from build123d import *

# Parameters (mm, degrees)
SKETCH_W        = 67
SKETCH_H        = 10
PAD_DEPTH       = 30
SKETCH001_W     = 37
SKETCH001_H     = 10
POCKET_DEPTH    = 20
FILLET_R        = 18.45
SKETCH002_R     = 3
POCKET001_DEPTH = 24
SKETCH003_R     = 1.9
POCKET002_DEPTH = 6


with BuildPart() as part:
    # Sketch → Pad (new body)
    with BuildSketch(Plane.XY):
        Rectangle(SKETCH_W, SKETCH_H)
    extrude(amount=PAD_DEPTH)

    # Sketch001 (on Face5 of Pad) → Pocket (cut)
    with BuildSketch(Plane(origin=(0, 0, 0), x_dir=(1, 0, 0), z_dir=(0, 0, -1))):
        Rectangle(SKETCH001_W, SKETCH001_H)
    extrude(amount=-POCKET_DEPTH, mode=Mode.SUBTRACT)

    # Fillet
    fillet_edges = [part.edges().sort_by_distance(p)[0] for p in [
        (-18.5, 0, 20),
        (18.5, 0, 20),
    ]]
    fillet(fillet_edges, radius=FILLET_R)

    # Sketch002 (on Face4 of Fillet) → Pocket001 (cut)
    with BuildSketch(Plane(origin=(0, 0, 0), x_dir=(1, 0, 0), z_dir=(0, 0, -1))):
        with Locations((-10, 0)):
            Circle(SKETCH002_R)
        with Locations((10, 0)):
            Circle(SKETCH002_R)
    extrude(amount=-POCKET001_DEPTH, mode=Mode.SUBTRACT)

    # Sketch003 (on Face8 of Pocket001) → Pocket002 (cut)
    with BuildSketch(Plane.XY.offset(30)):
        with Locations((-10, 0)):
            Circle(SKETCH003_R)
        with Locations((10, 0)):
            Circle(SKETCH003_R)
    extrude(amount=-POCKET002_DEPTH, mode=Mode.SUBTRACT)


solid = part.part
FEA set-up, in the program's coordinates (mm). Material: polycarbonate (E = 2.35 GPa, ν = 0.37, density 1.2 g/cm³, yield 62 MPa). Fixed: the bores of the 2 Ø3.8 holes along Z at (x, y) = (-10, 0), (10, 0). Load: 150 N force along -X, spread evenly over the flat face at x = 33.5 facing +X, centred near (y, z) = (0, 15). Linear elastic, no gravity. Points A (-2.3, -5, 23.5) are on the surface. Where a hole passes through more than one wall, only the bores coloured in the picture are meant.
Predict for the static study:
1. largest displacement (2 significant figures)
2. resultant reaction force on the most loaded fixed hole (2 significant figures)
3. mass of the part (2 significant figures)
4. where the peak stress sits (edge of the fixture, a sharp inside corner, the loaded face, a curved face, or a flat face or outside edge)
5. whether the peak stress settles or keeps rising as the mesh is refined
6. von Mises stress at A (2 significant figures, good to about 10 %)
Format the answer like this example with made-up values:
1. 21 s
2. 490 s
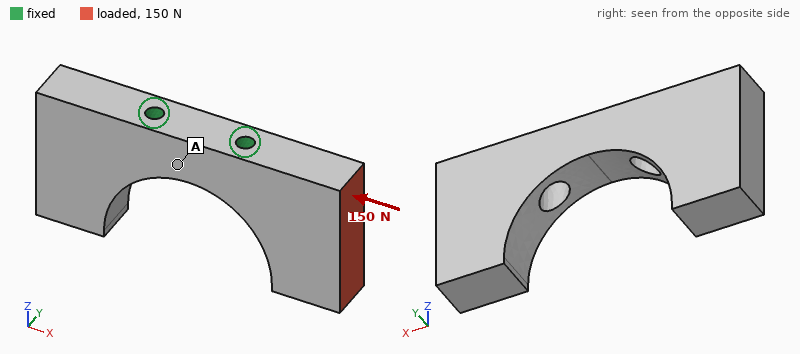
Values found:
1. 0.23 mm
2. 94 N
3. 16 g
4. edge of the fixture
5. keeps rising
6. 1.9 MPa
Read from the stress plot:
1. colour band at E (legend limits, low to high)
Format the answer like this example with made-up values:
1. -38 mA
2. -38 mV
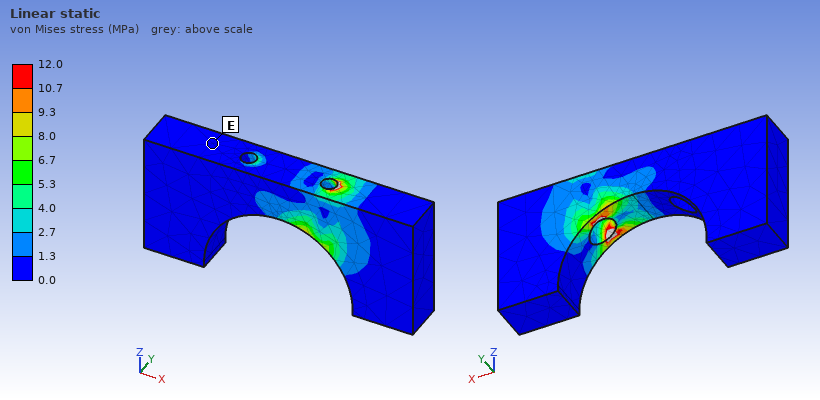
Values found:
1. 0.0 to 1.3 MPa
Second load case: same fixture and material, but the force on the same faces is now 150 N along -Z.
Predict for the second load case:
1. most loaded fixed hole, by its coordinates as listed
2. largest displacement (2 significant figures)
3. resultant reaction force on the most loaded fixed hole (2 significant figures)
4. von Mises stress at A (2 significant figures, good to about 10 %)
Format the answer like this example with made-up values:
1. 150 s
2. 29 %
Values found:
1. (10, 0)
2. 0.47 mm
3. 270 N
4. 3.3 MPa
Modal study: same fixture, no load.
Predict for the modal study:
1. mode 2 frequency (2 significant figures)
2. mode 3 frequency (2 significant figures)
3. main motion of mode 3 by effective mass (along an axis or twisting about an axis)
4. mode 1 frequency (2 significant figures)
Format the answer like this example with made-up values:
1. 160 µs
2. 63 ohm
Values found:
1. 1400 Hz
2. 1600 Hz
3. along X
4. 1400 Hz
